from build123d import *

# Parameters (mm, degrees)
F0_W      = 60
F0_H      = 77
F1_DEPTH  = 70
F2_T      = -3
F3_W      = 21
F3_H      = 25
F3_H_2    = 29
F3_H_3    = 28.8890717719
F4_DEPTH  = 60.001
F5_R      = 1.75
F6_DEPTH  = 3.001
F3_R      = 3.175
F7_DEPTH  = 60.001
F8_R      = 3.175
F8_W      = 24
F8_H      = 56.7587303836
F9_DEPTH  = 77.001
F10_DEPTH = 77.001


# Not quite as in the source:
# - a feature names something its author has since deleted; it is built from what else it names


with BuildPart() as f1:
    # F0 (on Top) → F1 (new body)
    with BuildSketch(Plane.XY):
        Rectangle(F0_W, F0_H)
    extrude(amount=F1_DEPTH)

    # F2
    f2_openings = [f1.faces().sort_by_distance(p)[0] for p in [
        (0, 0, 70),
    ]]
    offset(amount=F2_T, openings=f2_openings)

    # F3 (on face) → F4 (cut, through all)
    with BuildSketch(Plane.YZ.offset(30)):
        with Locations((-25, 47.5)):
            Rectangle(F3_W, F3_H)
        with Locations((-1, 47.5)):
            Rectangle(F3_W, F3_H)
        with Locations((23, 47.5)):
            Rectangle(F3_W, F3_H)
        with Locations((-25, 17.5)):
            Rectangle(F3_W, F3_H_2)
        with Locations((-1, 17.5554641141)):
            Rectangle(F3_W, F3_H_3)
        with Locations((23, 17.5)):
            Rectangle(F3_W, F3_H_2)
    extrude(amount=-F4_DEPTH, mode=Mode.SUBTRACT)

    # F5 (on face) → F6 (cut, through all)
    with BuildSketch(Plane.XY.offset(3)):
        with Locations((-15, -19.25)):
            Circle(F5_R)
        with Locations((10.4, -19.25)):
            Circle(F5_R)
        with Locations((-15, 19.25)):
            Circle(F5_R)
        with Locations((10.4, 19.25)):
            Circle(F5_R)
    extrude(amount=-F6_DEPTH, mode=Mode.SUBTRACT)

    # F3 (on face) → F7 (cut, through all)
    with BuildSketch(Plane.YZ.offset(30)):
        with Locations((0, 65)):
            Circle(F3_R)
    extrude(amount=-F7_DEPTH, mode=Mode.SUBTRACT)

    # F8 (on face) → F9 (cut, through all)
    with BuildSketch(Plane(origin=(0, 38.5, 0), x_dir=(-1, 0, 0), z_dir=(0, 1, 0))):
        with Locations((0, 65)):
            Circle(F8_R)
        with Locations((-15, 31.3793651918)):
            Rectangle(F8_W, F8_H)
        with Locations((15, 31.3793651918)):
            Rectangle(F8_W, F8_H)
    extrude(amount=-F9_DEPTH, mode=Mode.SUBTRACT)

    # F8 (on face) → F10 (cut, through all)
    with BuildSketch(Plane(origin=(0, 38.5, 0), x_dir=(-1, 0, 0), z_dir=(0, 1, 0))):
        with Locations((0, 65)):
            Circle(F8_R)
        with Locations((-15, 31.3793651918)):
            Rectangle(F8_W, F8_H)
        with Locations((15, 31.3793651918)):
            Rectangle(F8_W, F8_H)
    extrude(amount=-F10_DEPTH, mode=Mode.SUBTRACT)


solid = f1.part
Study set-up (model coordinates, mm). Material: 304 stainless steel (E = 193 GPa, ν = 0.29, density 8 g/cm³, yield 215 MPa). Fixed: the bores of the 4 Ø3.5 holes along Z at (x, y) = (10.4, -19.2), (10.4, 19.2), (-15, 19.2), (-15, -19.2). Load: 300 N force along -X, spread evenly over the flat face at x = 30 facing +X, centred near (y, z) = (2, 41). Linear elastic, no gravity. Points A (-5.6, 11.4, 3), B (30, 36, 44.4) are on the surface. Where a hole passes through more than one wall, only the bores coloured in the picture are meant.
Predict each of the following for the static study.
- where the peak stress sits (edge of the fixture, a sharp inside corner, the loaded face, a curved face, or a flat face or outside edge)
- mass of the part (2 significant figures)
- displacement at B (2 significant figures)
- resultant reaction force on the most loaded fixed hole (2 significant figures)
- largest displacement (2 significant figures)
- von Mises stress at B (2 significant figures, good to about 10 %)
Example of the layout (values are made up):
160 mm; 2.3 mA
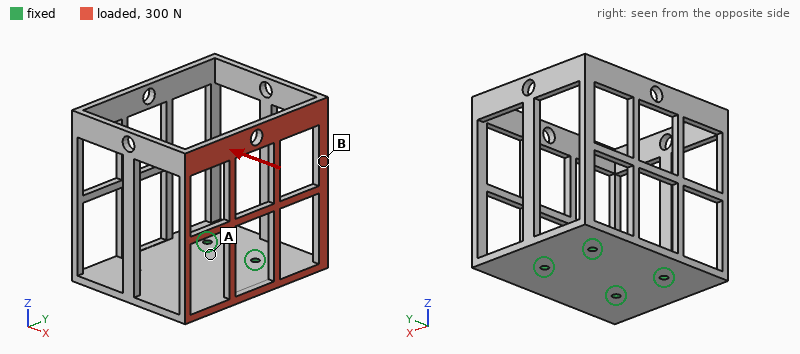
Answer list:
the loaded face; 230 g; 0.15 mm; 190 N; 0.25 mm; 37 MPa
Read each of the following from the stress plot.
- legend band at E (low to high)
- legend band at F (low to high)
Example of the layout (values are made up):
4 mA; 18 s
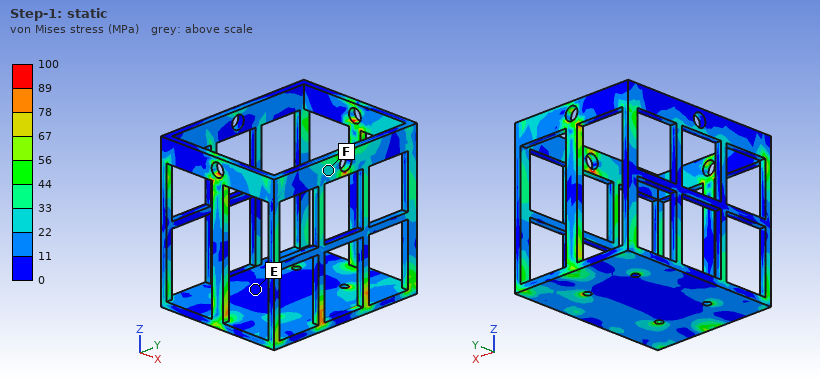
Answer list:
0 to 11 MPa; 22 to 33 MPa
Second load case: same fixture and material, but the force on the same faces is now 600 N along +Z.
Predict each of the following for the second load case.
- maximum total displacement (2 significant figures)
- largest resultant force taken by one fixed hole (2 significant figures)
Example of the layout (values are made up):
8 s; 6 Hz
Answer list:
89 µm; 430 N
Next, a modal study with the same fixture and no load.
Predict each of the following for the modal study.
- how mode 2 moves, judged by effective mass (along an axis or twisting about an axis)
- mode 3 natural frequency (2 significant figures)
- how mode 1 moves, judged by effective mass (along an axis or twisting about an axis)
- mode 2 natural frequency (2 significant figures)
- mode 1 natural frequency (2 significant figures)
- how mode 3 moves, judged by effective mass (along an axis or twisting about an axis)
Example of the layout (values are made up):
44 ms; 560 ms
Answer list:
along Y; 830 Hz; along X; 690 Hz; 570 Hz; twisting about Z
